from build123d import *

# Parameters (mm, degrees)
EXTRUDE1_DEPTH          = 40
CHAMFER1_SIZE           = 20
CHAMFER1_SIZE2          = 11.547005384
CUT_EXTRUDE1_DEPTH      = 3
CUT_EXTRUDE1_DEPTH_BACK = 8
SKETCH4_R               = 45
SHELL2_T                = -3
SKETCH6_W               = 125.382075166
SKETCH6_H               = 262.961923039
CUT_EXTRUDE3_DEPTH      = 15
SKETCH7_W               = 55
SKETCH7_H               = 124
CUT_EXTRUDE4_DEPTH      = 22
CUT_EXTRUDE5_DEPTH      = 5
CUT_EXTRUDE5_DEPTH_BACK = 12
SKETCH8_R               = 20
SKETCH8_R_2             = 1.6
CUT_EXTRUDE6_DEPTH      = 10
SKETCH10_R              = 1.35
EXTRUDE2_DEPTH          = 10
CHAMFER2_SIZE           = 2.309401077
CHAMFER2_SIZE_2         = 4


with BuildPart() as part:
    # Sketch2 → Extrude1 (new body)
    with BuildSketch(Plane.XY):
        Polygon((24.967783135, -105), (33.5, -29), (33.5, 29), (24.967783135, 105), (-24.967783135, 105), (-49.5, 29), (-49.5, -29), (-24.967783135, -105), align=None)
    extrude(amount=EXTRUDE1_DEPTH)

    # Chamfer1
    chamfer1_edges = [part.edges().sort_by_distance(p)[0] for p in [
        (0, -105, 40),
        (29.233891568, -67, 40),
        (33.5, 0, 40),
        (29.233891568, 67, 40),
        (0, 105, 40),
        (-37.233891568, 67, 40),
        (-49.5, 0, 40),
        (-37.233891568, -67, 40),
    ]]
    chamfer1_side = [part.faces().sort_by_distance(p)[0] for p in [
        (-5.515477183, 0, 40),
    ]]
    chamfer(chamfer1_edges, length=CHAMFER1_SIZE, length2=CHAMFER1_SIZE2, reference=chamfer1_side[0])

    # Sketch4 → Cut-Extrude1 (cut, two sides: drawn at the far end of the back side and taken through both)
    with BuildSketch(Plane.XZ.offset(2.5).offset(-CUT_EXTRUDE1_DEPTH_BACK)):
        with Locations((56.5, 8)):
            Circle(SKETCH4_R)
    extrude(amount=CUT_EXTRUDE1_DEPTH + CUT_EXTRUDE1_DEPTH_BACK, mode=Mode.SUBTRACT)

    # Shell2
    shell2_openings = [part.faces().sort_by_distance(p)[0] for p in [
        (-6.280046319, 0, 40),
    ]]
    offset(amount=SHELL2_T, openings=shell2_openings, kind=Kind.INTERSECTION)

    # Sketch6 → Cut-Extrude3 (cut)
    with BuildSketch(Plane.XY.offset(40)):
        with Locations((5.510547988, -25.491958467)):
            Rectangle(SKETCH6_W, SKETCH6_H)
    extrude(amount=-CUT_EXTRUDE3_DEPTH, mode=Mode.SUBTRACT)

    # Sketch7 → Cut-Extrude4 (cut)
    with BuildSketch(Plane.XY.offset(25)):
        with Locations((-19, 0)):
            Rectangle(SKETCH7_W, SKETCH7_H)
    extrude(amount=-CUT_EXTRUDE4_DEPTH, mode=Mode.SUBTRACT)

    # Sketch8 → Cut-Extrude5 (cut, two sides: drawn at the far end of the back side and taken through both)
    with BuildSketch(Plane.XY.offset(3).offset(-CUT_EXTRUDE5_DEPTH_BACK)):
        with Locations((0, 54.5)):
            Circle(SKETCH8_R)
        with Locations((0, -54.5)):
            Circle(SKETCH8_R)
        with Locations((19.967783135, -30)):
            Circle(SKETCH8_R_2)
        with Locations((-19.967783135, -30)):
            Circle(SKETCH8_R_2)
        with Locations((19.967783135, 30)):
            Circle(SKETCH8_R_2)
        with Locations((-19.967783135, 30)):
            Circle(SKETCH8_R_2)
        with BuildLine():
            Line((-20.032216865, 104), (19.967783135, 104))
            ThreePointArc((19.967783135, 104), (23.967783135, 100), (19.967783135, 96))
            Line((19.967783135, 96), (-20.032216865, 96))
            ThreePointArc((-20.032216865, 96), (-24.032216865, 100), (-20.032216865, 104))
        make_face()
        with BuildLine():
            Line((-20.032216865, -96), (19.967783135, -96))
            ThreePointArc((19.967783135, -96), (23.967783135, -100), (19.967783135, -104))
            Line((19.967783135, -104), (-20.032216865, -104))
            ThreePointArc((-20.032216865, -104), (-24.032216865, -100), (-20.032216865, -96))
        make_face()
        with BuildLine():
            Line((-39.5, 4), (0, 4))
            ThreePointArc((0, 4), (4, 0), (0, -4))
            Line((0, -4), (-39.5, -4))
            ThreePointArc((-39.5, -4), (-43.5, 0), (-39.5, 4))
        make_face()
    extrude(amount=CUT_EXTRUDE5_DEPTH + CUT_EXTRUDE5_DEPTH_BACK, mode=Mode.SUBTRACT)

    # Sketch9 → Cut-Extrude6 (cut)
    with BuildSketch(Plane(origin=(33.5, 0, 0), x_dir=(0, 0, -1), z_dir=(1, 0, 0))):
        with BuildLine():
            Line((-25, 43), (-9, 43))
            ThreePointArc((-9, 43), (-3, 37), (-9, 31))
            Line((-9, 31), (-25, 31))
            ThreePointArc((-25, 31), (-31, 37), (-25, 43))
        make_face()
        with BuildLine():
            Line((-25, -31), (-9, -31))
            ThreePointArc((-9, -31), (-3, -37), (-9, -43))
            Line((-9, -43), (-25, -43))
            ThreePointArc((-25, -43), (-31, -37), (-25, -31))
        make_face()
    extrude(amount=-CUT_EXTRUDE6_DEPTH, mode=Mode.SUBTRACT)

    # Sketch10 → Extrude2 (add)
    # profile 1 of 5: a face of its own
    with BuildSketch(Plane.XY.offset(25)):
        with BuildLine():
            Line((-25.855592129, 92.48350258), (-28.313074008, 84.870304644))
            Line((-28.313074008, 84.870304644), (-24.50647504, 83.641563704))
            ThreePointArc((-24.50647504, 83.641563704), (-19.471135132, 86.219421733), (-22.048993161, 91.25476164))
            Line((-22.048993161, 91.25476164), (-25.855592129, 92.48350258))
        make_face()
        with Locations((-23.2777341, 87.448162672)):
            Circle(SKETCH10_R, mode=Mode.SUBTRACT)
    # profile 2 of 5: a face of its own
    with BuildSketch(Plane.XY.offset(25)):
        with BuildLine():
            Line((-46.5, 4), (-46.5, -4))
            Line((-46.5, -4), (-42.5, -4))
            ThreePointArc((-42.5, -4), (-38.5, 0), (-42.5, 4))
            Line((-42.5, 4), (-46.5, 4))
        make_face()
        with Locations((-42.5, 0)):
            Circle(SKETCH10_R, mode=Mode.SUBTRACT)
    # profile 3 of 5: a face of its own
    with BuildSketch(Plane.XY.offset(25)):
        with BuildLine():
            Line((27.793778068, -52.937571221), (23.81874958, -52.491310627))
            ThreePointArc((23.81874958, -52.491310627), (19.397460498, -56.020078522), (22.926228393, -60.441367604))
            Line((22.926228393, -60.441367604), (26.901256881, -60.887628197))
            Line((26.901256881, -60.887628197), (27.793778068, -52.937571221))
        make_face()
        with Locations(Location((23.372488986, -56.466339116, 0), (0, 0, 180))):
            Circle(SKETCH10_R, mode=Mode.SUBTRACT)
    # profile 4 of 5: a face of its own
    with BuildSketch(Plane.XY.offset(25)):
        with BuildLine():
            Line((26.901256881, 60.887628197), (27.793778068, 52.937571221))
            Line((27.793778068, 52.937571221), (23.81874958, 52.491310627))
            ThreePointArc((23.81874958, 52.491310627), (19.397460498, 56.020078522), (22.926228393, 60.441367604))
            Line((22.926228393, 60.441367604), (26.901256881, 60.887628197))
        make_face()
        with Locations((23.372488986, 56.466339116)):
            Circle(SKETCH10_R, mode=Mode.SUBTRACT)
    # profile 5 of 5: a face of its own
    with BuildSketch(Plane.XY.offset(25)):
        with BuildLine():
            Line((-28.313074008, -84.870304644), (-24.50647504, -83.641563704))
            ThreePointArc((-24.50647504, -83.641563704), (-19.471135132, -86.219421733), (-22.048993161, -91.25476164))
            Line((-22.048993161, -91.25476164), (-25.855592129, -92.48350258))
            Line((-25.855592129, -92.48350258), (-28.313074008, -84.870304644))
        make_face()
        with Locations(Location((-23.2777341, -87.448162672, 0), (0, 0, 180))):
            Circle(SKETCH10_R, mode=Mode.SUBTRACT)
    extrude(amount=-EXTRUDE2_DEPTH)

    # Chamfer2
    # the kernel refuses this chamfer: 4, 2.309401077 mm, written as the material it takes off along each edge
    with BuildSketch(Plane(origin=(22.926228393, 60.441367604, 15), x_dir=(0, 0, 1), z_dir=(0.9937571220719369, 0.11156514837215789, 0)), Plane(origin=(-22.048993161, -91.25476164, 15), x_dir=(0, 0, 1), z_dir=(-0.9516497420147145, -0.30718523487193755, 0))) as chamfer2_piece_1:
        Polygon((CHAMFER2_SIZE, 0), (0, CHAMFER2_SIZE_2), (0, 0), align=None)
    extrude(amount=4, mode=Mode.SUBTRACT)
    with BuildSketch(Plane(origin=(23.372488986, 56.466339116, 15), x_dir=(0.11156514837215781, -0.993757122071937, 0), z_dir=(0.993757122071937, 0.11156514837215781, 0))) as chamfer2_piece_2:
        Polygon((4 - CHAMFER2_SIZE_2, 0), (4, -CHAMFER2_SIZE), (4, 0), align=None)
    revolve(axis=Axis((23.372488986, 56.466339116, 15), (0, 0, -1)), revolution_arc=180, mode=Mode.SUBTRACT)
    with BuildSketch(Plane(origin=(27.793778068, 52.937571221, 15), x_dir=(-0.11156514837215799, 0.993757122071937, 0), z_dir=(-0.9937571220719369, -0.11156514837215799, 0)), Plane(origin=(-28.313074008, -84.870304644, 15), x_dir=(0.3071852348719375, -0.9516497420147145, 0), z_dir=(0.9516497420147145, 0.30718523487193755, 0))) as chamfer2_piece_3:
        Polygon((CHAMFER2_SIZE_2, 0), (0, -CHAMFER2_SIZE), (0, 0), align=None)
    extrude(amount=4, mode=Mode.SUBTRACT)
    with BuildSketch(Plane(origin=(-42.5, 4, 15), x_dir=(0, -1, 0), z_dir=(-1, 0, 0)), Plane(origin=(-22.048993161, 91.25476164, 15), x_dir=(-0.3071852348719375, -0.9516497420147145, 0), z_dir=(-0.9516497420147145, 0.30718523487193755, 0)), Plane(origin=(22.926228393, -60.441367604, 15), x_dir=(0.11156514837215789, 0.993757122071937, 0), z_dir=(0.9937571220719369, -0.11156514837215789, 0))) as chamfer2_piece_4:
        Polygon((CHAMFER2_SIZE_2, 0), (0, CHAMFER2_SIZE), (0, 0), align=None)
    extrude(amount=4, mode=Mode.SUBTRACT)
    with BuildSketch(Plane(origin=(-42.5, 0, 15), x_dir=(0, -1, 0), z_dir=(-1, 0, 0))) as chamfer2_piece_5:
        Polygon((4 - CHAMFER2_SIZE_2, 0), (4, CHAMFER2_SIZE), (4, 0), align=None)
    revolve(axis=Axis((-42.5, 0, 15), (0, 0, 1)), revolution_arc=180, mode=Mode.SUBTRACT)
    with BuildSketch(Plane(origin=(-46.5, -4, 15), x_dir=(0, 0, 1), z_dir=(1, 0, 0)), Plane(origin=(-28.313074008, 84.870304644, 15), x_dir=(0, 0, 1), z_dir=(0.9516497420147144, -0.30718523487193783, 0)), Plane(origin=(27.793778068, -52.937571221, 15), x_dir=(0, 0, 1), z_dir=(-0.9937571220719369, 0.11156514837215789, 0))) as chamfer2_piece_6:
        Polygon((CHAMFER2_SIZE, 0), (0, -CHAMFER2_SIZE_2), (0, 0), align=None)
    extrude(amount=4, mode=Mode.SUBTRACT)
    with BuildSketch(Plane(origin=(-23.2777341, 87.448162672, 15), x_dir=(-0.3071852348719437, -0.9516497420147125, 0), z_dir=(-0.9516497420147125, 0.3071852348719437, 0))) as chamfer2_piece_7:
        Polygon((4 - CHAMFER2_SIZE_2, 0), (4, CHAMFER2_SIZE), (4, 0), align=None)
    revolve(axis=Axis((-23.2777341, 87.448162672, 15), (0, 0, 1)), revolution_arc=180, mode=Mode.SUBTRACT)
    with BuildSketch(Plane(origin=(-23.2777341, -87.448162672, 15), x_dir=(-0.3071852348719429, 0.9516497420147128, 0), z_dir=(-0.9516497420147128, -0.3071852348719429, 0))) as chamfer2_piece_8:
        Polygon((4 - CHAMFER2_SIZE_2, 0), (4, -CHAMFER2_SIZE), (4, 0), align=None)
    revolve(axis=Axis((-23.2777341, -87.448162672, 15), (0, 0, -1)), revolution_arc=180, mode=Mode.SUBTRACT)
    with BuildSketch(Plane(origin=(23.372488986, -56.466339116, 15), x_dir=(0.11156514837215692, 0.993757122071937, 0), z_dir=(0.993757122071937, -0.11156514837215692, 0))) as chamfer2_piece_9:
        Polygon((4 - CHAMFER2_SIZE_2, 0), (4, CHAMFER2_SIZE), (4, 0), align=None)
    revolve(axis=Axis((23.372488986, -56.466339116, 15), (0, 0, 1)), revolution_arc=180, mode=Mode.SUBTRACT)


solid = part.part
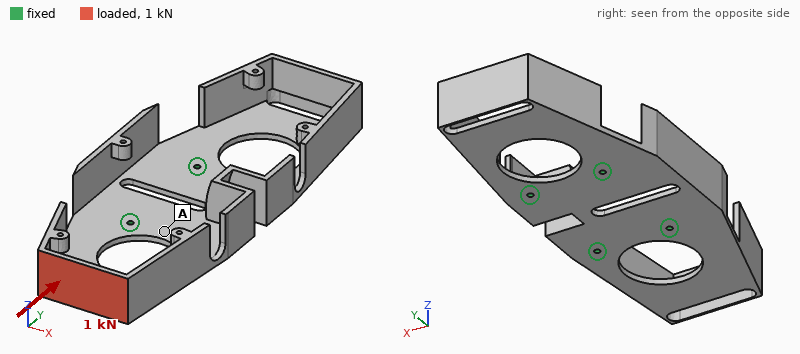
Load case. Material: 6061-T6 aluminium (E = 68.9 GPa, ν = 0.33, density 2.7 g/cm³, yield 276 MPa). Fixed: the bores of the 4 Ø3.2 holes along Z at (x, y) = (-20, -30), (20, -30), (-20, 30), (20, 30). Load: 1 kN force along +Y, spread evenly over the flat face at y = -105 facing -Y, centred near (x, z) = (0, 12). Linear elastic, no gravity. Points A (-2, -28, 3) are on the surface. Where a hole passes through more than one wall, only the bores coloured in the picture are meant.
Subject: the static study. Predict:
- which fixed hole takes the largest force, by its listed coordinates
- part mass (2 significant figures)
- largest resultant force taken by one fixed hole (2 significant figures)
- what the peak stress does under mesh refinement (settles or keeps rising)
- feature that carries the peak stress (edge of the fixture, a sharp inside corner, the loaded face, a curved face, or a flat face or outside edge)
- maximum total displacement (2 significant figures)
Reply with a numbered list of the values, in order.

1. (20, -30)
2. 180 g
3. 550 N
4. keeps rising
5. a sharp inside corner
6. 2.4 mm
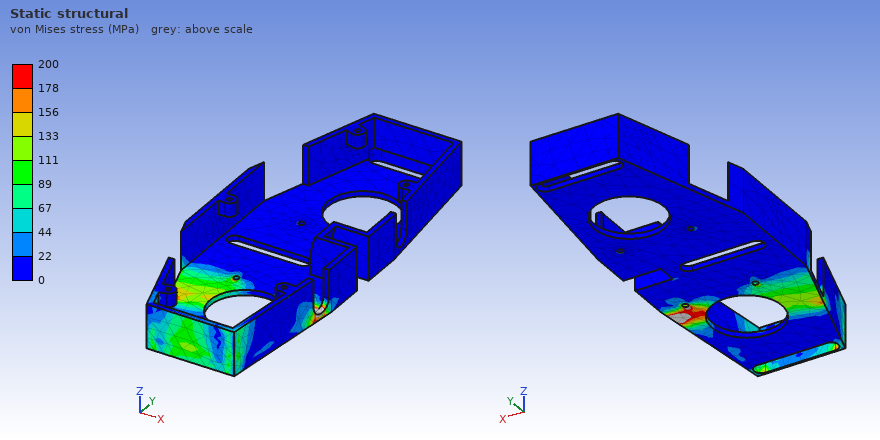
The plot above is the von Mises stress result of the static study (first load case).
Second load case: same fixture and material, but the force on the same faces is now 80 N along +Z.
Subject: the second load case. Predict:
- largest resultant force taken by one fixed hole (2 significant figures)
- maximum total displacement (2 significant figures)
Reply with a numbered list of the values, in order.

1. 82 N
2. 1.1 mm
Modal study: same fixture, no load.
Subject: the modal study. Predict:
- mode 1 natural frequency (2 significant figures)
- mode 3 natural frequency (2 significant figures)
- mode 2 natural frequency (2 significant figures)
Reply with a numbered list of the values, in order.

1. 300 Hz
2. 830 Hz
3. 300 Hz
